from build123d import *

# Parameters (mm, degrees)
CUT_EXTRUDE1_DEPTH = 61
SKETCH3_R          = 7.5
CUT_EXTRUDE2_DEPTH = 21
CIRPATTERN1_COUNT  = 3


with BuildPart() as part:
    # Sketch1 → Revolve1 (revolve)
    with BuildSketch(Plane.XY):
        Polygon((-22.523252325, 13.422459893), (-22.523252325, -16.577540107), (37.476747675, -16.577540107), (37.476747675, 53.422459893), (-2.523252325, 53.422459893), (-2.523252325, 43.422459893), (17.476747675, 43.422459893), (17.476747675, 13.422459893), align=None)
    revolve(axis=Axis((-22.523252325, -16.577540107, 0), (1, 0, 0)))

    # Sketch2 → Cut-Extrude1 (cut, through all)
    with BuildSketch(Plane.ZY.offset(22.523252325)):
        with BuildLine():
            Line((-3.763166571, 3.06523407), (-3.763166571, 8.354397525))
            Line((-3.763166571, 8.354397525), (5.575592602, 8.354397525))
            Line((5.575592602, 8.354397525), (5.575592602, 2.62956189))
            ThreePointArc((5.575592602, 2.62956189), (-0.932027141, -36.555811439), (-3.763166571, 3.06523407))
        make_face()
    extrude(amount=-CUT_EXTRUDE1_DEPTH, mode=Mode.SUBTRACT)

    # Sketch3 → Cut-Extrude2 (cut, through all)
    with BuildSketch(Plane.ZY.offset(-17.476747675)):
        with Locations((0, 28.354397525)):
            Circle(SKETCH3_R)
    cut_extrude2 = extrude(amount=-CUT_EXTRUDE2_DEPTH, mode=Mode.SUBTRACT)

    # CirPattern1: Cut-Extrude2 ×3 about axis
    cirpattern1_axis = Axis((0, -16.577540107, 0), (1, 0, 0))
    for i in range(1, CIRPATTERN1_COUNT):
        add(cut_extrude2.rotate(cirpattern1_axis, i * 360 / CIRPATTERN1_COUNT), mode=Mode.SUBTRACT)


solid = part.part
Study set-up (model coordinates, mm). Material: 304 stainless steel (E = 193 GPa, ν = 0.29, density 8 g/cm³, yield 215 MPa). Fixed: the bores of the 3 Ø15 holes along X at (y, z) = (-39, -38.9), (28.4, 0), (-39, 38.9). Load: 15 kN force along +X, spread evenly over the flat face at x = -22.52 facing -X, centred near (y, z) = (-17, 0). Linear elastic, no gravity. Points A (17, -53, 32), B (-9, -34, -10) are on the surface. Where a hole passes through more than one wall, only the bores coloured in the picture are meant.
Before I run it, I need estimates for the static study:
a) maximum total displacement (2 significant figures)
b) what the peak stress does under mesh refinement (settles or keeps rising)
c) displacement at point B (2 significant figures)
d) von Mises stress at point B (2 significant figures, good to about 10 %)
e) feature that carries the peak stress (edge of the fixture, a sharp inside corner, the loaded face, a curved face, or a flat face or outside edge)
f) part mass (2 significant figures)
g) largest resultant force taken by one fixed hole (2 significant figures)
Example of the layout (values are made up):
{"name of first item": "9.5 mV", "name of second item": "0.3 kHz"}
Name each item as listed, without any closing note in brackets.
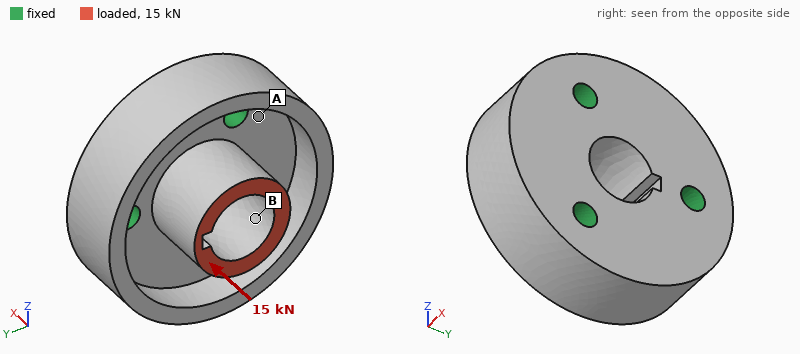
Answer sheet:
{"maximum total displacement": "4.4 µm", "what the peak stress does under mesh refinement": "keeps rising", "displacement at point B": "3.6 µm", "von Mises stress at point B": "11 MPa", "feature that carries the peak stress": "edge of the fixture", "part mass": "3.3 kg", "largest resultant force taken by one fixed hole": "5.2 kN"}
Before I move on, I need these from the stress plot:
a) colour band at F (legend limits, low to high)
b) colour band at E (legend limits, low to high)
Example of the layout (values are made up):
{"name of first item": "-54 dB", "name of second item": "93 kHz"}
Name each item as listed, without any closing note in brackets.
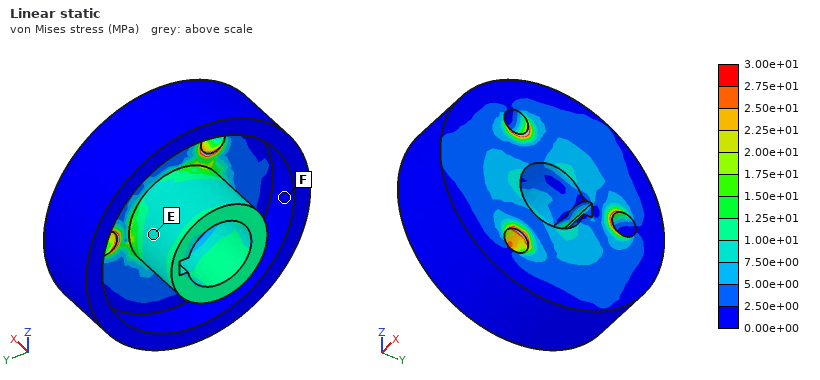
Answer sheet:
{"colour band at F": "0.00e+00 to 2.50e+00 MPa", "colour band at E": "7.50e+00 to 1.00e+01 MPa"}
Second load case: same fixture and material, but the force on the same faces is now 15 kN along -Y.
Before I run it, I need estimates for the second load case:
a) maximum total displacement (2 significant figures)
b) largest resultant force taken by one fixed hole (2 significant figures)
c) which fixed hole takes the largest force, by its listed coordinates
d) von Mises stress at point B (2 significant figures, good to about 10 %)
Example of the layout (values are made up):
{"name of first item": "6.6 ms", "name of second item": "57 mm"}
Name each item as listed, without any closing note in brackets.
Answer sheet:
{"maximum total displacement": "31 µm", "largest resultant force taken by one fixed hole": "12 kN", "which fixed hole takes the largest force, by its listed coordinates": "(28.4, 0)", "von Mises stress at point B": "29 MPa"}
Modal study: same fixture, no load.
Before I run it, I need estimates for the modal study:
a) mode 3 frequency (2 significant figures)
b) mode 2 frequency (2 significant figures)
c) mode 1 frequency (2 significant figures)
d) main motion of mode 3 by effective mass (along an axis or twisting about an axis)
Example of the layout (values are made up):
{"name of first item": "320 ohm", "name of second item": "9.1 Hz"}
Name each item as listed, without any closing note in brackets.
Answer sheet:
{"mode 3 frequency": "7400 Hz", "mode 2 frequency": "5600 Hz", "mode 1 frequency": "5600 Hz", "main motion of mode 3 by effective mass": "along X"}
